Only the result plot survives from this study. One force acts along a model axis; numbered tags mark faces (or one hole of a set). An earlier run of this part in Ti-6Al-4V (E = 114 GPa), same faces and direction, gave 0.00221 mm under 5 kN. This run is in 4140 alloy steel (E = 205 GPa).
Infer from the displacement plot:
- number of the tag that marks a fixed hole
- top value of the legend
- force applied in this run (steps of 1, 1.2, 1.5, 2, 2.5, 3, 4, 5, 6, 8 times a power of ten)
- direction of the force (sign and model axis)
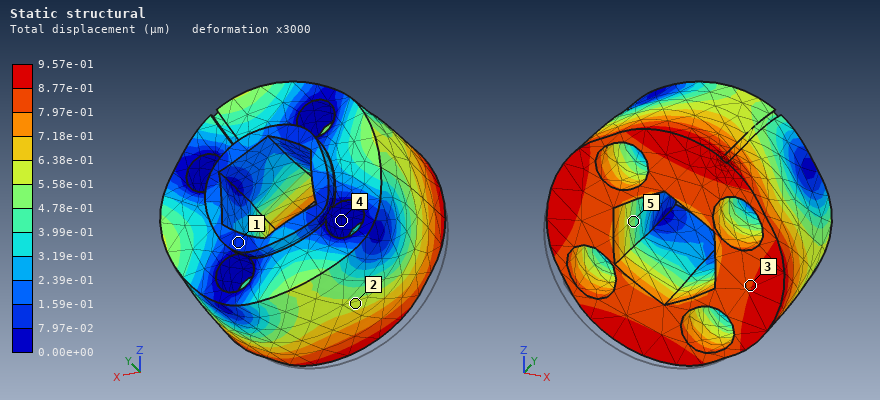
4
9.57e-01 µm
4 kN
+Y
